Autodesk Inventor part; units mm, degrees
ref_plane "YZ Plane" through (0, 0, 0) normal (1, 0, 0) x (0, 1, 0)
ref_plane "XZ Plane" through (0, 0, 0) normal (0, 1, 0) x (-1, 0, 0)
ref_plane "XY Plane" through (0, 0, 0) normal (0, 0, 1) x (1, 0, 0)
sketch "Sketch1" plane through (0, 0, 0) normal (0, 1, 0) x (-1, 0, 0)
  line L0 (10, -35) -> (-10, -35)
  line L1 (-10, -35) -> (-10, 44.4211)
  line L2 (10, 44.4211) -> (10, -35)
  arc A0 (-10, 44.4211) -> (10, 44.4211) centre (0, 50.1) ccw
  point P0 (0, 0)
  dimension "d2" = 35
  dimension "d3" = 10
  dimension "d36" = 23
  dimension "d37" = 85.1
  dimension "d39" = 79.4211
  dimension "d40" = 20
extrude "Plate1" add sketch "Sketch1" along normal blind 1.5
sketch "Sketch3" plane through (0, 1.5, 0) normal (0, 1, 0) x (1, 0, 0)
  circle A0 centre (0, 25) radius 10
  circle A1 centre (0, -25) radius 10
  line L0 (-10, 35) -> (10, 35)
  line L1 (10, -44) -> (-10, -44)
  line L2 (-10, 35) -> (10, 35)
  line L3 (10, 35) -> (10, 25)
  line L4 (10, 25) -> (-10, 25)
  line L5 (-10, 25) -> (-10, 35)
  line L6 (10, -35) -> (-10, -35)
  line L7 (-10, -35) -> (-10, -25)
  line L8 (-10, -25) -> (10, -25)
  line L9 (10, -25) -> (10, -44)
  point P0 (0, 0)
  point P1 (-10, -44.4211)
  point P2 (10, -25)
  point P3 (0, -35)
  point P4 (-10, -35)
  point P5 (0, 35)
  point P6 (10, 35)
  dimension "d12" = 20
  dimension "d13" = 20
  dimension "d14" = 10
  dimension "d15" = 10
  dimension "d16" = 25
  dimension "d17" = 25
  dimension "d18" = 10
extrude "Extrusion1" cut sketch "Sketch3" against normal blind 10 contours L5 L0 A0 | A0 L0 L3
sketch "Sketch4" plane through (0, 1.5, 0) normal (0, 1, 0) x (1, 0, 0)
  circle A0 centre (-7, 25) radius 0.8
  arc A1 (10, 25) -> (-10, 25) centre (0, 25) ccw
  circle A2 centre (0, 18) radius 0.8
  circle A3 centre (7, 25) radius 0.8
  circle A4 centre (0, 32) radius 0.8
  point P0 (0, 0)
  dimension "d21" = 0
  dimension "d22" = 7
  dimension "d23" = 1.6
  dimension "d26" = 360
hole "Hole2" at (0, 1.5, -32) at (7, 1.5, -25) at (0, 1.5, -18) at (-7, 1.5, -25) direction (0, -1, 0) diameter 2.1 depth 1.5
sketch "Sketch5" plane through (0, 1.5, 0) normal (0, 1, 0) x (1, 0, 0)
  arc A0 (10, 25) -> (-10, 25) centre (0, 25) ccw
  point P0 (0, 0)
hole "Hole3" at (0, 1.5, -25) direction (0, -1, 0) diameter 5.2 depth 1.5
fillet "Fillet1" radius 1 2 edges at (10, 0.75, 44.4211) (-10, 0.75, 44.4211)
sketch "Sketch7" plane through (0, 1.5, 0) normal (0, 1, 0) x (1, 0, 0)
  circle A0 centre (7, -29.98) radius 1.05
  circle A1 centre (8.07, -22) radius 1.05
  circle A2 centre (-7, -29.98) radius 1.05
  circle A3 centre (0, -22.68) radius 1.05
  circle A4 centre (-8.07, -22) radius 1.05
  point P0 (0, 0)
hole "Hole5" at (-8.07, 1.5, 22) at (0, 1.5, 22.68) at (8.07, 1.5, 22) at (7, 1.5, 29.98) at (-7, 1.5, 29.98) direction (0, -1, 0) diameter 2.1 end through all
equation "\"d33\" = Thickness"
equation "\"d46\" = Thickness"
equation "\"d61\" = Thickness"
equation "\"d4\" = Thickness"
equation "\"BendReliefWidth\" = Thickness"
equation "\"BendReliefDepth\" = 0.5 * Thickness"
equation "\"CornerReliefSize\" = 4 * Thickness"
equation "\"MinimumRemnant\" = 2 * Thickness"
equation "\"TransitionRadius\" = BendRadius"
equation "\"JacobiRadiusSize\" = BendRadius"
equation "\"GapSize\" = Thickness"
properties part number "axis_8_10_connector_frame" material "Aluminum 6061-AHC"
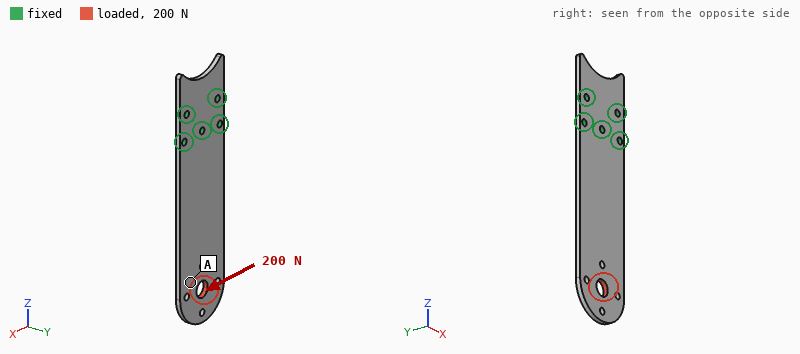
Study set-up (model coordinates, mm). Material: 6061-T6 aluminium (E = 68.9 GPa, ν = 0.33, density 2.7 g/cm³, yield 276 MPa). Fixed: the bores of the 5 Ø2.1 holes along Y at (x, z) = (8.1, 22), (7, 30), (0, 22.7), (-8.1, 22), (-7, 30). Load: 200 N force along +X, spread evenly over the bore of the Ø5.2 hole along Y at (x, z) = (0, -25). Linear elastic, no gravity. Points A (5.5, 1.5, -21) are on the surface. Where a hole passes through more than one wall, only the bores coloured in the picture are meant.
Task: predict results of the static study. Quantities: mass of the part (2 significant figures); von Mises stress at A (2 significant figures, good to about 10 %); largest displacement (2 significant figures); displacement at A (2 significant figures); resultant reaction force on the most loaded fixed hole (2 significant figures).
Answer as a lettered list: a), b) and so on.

a) 5.7 g
b) 12 MPa
c) 0.15 mm
d) 0.10 mm
e) 540 N
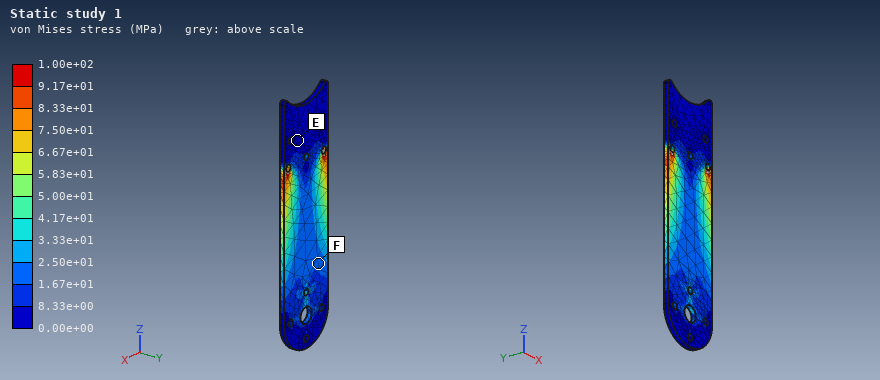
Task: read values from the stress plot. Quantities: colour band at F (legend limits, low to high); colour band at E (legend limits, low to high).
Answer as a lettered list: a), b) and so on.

a) 1.67e+01 to 2.50e+01 MPa
b) 0.00e+00 to 8.33e+00 MPa
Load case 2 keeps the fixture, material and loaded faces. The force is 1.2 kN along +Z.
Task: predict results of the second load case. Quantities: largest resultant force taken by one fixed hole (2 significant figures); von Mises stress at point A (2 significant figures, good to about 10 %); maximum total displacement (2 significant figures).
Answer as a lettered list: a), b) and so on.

a) 380 N
b) 47 MPa
c) 34 µm
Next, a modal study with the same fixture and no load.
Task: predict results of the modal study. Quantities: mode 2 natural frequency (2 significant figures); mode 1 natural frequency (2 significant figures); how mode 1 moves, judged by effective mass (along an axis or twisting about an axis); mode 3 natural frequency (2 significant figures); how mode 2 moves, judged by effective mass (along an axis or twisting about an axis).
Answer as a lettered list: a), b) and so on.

a) 2400 Hz
b) 430 Hz
c) along Y
d) 2600 Hz
e) twisting about Z
